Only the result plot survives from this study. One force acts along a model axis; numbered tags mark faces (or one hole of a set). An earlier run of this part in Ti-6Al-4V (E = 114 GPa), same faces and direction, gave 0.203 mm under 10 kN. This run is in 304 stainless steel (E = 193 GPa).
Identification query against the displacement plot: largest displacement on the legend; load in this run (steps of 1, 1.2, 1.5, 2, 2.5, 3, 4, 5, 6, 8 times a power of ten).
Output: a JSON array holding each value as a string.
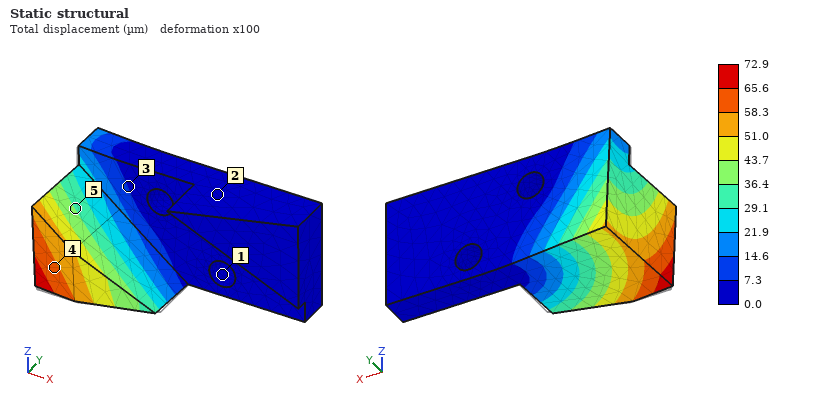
["72.9 µm", "6 kN"]
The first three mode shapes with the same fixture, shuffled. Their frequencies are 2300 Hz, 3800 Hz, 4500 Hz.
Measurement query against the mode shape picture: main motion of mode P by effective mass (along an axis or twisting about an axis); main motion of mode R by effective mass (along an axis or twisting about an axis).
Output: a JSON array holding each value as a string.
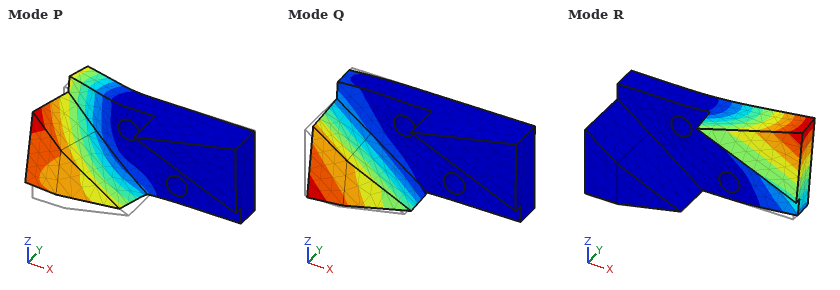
["along Z", "along Y"]
